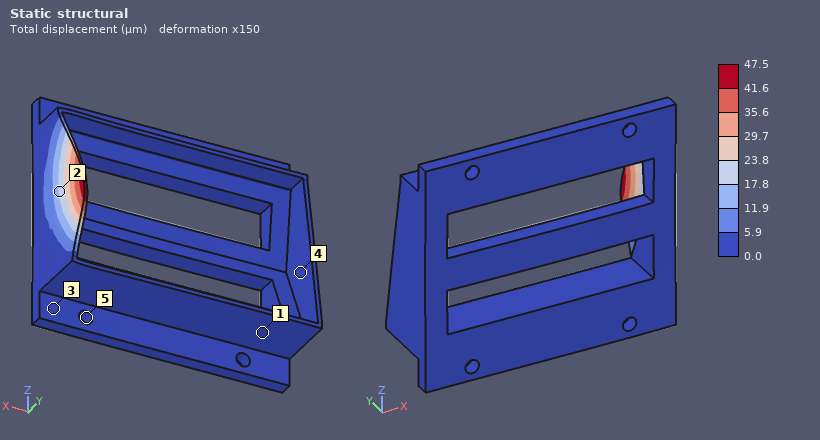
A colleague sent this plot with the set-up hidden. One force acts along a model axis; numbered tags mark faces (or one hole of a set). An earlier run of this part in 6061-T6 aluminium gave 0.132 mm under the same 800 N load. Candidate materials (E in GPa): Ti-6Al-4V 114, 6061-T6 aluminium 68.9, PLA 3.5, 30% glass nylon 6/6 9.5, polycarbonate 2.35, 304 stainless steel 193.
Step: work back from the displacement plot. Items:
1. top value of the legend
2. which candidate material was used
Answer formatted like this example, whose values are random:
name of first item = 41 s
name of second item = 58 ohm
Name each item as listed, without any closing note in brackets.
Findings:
top value of the legend = 47.5 µm
which candidate material was used = 304 stainless steel
